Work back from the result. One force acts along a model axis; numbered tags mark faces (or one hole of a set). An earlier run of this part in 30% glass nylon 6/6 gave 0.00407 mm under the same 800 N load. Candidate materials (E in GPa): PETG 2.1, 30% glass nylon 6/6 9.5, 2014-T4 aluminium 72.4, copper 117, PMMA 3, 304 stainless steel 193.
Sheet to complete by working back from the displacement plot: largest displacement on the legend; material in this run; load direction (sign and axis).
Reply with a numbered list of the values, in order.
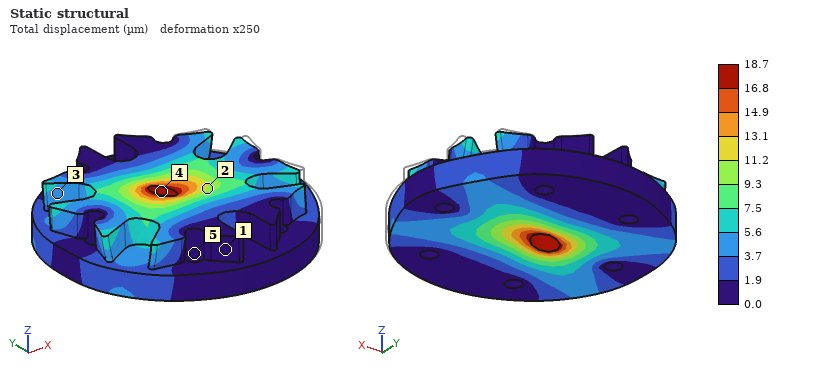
1. 18.7 µm
2. PETG
3. -X
